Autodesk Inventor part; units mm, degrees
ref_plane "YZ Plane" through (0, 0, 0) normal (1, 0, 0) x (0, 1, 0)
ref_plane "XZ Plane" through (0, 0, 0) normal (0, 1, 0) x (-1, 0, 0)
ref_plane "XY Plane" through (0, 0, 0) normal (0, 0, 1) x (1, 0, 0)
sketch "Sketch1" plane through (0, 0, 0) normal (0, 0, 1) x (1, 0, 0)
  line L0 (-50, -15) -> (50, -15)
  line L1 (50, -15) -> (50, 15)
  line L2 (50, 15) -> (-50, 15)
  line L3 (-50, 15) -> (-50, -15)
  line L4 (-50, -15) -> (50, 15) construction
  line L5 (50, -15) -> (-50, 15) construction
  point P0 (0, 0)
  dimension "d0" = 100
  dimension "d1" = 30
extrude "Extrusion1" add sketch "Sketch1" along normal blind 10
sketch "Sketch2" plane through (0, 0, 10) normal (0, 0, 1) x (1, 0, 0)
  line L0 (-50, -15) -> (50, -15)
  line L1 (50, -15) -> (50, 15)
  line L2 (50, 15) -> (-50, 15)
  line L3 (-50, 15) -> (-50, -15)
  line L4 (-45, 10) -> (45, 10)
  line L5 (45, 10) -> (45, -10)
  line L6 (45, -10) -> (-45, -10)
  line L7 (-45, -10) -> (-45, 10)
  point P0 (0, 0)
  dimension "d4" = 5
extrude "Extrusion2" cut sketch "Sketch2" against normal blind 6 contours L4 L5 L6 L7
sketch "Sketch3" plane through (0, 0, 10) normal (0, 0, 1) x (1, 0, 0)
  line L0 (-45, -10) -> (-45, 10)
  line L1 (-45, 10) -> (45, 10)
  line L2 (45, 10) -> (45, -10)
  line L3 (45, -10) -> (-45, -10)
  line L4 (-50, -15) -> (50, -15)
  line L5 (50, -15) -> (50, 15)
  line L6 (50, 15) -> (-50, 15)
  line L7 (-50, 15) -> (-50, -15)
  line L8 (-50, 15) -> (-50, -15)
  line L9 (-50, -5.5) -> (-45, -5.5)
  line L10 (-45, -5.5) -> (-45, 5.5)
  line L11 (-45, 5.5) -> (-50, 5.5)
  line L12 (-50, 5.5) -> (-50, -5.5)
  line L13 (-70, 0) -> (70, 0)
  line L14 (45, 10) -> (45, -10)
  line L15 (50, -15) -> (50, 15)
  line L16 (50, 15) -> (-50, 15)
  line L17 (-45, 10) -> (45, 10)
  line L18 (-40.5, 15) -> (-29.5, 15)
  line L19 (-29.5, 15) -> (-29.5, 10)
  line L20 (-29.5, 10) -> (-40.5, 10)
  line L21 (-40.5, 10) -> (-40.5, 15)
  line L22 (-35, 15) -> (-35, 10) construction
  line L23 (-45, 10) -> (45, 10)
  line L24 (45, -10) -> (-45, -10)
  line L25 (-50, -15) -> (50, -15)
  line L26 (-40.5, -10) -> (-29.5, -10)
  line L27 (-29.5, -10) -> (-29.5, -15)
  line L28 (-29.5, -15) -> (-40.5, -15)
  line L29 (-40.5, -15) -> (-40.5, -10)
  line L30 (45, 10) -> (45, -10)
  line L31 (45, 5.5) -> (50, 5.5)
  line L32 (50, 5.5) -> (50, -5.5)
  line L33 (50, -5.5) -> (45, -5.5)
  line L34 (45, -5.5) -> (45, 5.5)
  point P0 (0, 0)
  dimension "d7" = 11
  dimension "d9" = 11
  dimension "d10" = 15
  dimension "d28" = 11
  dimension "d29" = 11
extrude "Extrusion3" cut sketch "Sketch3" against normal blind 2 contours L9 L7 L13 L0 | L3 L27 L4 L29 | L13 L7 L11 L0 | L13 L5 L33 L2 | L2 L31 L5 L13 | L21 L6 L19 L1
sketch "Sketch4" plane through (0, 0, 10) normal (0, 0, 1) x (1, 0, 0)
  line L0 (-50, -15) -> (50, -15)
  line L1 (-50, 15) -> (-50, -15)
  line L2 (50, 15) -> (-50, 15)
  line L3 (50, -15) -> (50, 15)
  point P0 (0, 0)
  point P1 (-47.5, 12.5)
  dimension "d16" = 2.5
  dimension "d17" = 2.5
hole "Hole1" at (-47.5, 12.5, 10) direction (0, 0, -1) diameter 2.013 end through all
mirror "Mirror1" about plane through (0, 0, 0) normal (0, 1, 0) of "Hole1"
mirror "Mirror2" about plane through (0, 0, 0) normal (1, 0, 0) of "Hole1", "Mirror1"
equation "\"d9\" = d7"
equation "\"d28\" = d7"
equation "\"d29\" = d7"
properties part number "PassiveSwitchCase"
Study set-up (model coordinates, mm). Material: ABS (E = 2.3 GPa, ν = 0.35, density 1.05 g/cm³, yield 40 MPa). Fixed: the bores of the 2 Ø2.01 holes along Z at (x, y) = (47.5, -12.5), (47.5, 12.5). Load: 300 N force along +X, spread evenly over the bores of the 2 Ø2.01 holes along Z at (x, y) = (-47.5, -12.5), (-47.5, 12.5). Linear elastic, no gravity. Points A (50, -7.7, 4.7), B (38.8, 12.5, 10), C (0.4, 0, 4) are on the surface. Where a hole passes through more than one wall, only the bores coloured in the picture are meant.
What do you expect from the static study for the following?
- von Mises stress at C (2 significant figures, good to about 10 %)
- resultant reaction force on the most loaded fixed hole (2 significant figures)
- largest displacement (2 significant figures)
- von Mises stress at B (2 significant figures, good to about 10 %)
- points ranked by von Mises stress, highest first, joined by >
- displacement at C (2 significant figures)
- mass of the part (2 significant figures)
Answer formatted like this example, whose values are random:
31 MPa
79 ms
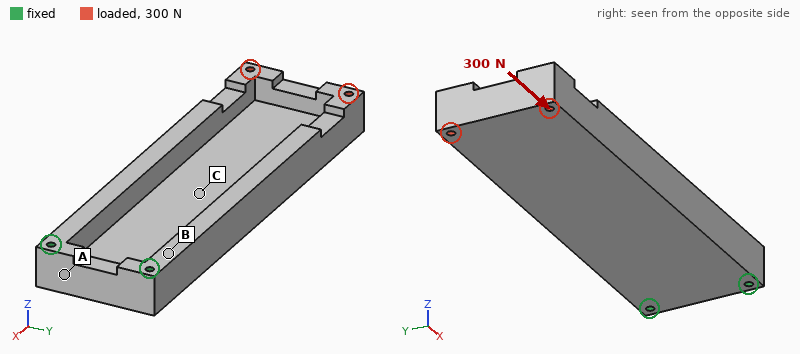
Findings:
1.7 MPa
150 N
0.62 mm
3.3 MPa
B > C > A
0.12 mm
20 g
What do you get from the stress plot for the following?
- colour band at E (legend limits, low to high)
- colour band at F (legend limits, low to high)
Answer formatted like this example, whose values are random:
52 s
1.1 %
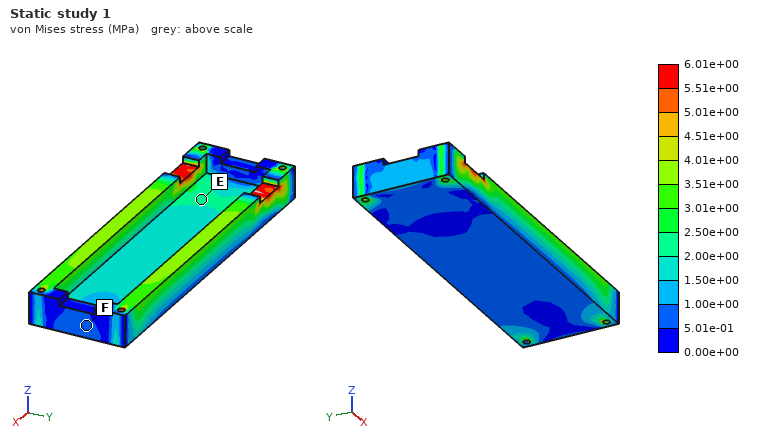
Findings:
2.00e+00 to 2.50e+00 MPa
5.01e-01 to 1.00e+00 MPa
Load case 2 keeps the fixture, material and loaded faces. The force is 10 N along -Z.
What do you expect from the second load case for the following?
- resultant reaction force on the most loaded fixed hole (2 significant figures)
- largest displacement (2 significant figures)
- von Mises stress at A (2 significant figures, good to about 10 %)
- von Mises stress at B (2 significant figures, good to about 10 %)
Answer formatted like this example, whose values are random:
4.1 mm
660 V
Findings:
15 N
1.1 mm
1.1 MPa
4.2 MPa
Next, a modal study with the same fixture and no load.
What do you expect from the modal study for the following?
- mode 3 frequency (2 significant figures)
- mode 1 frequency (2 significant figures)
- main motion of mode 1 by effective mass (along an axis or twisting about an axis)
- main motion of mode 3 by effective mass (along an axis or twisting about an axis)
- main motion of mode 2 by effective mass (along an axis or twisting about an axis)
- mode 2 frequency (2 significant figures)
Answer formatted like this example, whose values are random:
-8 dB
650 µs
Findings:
890 Hz
220 Hz
along Z
along Y
along Y
590 Hz
